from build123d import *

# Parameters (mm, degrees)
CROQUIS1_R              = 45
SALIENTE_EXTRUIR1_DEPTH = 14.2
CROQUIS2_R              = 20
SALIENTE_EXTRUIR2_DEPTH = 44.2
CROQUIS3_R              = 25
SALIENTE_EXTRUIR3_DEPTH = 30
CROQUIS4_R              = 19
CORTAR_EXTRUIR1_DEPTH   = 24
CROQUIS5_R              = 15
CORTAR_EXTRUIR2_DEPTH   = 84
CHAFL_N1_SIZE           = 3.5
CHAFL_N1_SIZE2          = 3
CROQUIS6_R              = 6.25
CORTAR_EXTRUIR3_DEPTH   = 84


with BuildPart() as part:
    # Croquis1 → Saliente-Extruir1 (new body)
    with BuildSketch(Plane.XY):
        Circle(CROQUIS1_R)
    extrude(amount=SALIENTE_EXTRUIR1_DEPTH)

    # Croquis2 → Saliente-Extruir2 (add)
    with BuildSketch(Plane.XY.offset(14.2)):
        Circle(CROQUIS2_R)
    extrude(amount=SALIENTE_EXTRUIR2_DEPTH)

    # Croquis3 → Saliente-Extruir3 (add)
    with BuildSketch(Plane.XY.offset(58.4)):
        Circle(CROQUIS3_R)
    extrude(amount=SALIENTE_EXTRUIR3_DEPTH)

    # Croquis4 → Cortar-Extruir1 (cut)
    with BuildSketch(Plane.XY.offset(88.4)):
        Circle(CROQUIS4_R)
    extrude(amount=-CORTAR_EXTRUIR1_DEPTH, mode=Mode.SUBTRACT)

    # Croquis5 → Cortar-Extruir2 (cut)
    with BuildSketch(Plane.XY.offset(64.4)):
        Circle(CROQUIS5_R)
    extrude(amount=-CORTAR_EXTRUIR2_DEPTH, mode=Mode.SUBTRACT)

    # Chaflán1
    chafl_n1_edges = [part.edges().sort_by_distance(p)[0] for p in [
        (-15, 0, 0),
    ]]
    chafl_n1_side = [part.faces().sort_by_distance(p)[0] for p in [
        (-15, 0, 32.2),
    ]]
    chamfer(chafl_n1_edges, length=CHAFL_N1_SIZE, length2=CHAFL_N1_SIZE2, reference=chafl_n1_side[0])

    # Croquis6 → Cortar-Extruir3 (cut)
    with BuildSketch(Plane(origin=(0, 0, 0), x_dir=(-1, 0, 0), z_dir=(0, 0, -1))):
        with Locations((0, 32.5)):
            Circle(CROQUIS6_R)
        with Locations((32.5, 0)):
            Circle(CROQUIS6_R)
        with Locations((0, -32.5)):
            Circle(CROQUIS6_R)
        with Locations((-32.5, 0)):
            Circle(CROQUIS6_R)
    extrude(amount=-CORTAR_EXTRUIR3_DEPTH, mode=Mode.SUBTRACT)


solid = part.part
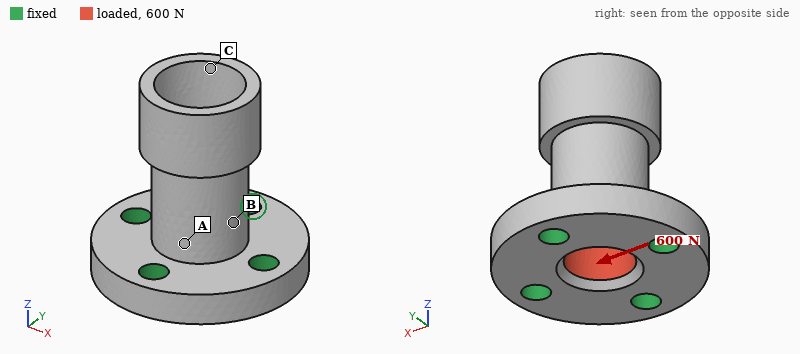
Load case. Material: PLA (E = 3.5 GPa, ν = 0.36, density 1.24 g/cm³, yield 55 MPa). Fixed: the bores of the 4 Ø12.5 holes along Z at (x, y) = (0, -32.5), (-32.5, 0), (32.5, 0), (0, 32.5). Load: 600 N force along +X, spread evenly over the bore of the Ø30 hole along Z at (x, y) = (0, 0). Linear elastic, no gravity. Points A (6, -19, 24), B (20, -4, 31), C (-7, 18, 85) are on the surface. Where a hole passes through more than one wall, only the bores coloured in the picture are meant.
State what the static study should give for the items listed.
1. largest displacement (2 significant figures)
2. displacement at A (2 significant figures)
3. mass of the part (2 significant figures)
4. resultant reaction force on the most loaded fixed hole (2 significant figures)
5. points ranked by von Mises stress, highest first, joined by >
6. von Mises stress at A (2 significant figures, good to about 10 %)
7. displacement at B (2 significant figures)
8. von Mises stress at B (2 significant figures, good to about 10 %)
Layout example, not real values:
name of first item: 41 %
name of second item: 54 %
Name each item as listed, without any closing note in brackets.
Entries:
largest displacement: 0.12 mm
displacement at A: 0.021 mm
mass of the part: 150 g
resultant reaction force on the most loaded fixed hole: 340 N
points ranked by von Mises stress, highest first, joined by >: A > B > C
von Mises stress at A: 1.7 MPa
displacement at B: 0.042 mm
von Mises stress at B: 1.1 MPa
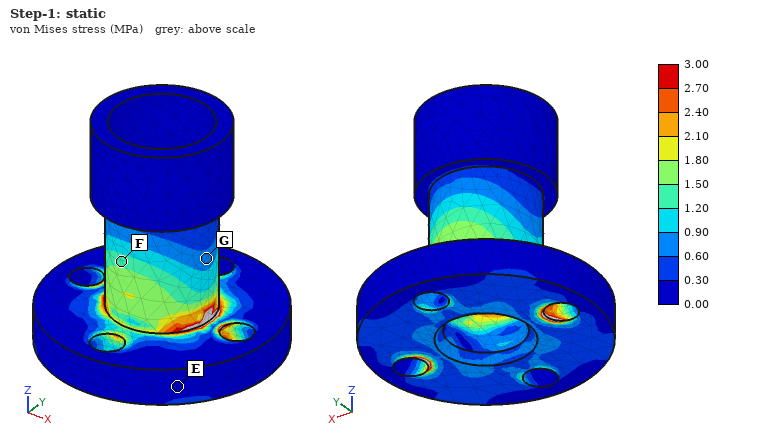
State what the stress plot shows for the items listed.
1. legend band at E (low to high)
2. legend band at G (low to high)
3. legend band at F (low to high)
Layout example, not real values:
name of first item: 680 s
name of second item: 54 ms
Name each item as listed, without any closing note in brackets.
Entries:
legend band at E: 0.00 to 0.30 MPa
legend band at G: 0.60 to 0.90 MPa
legend band at F: 1.20 to 1.50 MPa
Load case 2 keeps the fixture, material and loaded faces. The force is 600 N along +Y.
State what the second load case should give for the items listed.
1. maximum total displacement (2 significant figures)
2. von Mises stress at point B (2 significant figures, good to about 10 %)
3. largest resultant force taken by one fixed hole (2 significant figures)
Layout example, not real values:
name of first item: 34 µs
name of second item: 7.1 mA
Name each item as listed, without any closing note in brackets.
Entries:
maximum total displacement: 0.12 mm
von Mises stress at point B: 1.8 MPa
largest resultant force taken by one fixed hole: 340 N
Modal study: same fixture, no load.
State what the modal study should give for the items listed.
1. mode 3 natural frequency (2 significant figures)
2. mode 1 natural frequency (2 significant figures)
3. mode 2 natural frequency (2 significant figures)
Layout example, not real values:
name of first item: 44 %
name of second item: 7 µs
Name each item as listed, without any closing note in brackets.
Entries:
mode 3 natural frequency: 2300 Hz
mode 1 natural frequency: 1100 Hz
mode 2 natural frequency: 1100 Hz
